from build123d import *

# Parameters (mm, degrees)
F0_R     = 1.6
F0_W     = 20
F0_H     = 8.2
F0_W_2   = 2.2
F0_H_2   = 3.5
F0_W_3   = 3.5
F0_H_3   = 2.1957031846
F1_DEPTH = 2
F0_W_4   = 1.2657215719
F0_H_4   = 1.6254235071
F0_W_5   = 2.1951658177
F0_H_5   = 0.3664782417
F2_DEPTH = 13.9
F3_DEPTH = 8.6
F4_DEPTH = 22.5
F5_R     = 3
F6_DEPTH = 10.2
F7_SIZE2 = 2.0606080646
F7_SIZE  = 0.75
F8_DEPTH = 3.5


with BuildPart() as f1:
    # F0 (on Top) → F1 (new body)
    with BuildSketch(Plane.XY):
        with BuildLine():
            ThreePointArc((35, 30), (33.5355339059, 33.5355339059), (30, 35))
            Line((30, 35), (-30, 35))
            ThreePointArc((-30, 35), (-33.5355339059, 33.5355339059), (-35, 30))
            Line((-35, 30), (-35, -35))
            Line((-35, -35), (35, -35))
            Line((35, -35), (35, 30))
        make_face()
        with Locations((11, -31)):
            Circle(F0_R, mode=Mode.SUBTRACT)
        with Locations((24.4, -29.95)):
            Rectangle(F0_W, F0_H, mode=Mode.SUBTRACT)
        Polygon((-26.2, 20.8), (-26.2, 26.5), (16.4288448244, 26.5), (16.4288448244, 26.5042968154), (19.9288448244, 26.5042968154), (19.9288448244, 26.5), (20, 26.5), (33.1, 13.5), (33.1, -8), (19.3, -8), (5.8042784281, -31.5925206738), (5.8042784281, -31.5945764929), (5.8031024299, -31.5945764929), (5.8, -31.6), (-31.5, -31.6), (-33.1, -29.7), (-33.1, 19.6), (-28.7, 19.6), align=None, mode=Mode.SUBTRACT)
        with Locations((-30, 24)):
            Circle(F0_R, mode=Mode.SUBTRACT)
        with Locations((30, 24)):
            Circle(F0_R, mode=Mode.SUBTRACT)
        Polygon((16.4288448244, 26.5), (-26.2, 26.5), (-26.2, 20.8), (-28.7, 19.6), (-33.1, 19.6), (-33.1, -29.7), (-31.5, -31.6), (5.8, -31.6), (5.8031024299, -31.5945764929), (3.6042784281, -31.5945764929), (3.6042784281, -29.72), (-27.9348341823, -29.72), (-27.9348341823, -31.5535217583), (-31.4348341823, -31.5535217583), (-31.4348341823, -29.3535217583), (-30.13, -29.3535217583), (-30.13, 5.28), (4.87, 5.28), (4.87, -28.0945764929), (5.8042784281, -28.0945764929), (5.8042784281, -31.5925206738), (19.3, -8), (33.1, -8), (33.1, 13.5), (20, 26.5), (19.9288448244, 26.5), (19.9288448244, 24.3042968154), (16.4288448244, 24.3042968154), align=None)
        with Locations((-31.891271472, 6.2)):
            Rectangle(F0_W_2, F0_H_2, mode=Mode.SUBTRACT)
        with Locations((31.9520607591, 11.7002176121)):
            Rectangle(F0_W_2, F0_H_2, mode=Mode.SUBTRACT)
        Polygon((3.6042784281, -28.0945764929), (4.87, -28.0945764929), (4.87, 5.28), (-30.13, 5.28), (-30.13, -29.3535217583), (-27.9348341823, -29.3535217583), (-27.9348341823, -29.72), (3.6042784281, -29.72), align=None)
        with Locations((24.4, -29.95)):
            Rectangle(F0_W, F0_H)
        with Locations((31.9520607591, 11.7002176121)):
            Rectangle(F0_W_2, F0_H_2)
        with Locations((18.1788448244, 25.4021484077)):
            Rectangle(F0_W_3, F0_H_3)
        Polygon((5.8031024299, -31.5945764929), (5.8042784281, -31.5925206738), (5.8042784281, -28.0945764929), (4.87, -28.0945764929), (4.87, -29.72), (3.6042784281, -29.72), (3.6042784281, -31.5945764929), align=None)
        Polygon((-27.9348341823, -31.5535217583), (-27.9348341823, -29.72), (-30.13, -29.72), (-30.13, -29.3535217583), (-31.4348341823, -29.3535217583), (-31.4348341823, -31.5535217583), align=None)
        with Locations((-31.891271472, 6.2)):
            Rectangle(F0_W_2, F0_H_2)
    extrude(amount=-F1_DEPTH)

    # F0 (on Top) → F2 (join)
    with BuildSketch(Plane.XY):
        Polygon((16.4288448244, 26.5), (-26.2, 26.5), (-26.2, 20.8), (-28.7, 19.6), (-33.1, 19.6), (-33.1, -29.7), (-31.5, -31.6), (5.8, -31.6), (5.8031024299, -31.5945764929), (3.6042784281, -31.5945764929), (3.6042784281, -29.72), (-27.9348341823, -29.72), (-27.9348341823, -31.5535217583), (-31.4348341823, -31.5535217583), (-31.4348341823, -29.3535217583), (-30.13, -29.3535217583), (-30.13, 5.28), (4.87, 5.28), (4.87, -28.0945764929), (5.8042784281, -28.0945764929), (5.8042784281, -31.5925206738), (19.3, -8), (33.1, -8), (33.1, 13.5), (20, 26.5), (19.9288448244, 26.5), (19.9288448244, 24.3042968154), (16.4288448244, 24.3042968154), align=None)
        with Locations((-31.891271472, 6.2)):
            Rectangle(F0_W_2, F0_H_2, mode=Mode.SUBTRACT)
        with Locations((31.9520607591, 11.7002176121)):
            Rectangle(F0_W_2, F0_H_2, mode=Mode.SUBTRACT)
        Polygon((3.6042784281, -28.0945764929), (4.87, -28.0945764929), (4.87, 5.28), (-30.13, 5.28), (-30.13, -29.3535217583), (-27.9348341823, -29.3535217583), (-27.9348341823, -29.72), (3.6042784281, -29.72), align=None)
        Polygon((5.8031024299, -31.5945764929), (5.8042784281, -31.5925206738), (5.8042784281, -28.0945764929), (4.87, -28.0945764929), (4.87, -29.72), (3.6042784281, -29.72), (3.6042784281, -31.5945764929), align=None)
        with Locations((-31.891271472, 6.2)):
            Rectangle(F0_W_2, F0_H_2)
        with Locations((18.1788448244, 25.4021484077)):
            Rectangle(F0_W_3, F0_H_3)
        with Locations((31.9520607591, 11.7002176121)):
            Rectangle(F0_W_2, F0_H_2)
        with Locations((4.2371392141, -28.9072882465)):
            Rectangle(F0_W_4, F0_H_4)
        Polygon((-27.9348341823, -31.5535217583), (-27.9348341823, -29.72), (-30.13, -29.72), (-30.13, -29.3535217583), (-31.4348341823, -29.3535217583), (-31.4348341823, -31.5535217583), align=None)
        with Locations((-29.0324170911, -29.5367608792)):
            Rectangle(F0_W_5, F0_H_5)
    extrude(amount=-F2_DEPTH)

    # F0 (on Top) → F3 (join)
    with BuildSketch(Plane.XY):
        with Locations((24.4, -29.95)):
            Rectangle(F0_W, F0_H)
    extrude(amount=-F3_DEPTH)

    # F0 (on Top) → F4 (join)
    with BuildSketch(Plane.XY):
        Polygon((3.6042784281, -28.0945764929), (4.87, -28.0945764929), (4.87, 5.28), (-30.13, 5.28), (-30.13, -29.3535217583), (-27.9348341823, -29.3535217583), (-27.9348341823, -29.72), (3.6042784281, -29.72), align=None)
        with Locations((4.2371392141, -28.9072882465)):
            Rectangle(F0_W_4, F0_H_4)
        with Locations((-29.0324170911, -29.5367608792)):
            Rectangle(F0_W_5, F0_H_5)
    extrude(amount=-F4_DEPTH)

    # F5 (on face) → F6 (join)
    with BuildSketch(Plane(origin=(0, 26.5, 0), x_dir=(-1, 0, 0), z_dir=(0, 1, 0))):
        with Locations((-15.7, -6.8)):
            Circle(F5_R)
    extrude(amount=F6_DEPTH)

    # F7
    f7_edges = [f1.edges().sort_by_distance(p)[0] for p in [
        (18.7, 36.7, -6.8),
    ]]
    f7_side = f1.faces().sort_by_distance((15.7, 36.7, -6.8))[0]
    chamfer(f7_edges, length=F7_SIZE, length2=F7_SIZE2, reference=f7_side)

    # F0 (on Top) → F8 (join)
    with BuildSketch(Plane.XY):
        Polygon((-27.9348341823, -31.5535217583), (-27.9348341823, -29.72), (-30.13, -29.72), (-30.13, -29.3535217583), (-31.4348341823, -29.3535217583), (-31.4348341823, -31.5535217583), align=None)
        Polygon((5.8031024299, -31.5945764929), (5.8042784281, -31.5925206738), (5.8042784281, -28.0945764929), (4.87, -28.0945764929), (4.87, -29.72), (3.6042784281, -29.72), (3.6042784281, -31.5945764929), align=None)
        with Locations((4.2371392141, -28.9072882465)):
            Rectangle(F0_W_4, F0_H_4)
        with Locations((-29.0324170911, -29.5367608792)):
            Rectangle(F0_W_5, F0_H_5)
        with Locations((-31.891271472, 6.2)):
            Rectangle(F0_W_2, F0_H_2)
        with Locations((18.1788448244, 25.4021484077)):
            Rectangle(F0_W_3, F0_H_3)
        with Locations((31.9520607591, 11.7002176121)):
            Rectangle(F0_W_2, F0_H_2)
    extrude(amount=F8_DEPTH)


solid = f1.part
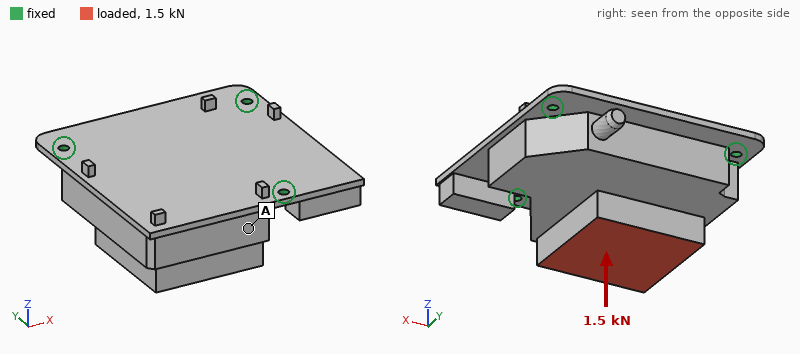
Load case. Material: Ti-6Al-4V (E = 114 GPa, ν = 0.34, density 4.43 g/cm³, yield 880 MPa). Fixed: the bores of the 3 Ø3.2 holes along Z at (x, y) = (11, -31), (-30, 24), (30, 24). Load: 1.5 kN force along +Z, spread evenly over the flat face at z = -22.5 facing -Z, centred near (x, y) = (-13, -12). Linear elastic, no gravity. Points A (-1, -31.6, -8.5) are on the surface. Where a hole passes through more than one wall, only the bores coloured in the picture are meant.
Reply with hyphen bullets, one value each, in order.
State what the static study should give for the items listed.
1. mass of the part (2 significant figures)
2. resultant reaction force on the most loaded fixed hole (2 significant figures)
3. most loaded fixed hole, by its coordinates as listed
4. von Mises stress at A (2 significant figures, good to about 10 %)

- 270 g
- 1.2 kN
- (11, -31)
- 12 MPa
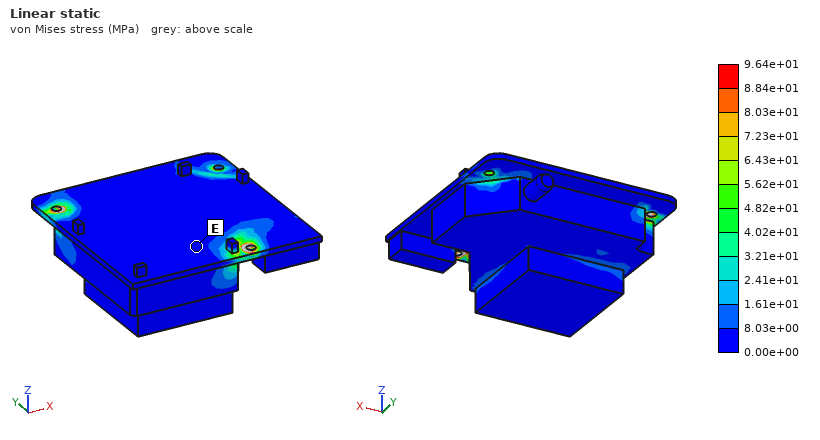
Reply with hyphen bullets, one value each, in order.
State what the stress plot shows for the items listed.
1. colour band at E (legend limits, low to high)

- 0.00e+00 to 8.03e+00 MPa
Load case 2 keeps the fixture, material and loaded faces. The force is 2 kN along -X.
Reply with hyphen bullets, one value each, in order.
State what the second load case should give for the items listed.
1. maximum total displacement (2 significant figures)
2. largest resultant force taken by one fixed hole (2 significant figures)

- 35 µm
- 1.3 kN
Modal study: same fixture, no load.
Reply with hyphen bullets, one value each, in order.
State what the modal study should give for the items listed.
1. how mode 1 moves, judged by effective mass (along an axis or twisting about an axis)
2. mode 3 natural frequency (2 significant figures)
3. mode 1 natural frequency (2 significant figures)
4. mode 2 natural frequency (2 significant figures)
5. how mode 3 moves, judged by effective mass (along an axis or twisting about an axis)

- along Z
- 4600 Hz
- 3100 Hz
- 3800 Hz
- along Z
